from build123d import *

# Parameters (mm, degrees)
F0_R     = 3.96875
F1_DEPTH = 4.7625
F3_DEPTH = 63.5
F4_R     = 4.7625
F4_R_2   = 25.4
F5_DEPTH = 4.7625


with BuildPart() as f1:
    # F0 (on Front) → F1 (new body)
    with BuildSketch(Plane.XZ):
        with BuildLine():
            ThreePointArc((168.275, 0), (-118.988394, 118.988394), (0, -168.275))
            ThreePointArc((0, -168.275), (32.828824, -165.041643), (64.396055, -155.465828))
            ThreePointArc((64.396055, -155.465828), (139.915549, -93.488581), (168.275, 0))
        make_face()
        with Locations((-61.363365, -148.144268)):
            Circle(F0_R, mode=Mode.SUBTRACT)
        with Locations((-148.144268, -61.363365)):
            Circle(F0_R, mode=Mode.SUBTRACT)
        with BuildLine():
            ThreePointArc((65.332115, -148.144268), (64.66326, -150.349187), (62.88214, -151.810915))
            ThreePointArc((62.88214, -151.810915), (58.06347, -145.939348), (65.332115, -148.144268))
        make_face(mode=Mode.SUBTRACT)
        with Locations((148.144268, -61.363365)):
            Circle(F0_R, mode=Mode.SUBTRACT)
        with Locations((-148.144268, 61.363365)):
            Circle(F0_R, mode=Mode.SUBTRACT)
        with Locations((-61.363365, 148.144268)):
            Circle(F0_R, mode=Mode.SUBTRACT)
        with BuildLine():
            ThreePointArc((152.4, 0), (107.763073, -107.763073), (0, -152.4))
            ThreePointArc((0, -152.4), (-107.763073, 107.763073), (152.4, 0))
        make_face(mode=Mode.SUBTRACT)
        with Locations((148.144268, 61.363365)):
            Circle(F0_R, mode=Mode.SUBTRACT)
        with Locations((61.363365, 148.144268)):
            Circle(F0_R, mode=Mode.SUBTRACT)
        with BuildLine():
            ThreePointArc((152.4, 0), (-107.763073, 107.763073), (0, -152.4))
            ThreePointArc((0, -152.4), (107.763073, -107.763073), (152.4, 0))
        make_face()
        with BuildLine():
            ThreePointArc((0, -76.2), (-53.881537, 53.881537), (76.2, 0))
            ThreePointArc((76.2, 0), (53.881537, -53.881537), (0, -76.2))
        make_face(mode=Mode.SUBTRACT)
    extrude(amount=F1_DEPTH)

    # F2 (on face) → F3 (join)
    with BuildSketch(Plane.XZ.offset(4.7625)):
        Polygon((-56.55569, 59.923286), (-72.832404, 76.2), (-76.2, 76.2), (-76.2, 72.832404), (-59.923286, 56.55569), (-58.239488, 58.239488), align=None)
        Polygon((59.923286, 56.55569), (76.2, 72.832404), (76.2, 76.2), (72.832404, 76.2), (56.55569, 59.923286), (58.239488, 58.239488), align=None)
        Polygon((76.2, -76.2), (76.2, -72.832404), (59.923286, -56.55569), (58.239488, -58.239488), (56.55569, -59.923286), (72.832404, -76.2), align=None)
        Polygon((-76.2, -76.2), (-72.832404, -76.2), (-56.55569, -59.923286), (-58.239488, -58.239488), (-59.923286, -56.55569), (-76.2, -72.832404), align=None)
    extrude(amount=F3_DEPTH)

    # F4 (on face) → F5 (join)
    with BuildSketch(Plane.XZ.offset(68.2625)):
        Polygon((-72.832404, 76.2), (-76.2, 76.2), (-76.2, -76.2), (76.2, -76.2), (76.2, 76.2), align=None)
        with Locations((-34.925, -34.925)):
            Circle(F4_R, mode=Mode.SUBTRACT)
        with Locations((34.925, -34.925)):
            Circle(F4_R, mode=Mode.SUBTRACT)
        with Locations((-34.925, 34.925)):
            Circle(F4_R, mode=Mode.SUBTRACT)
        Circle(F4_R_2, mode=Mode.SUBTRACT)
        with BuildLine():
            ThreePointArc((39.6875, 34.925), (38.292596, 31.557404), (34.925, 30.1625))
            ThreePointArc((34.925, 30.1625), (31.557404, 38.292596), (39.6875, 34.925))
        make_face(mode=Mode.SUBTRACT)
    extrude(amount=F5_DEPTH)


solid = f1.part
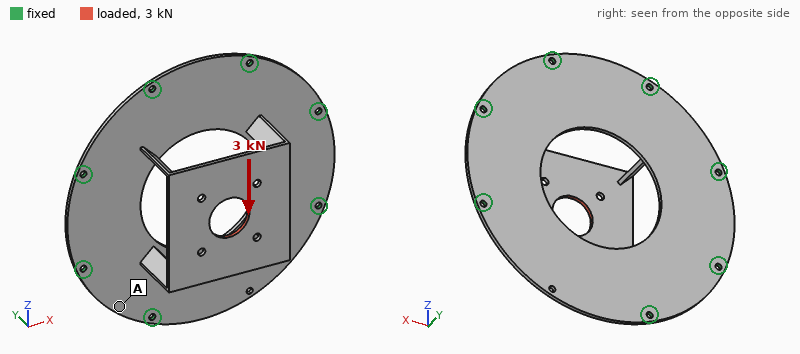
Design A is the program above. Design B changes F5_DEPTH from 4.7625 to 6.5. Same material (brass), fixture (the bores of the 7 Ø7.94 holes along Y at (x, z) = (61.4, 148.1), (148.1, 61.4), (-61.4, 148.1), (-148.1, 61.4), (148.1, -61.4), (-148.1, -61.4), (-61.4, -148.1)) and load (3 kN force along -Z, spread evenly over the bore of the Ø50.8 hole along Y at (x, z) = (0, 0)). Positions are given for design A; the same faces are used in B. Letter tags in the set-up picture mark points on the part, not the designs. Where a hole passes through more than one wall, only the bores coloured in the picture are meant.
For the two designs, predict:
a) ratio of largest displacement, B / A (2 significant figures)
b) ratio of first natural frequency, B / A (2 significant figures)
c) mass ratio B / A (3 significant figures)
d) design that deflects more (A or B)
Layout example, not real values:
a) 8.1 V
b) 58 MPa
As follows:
a) 0.79
b) 0.97
c) 1.08
d) A
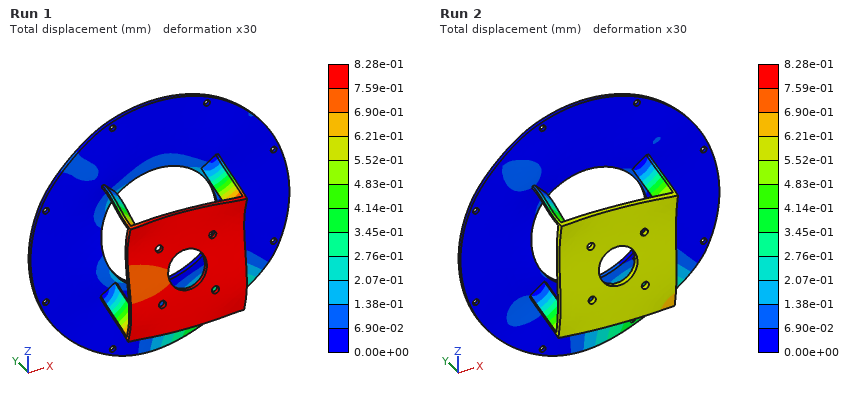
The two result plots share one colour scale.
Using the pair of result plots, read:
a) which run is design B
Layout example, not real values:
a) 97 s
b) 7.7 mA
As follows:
a) Run 2
